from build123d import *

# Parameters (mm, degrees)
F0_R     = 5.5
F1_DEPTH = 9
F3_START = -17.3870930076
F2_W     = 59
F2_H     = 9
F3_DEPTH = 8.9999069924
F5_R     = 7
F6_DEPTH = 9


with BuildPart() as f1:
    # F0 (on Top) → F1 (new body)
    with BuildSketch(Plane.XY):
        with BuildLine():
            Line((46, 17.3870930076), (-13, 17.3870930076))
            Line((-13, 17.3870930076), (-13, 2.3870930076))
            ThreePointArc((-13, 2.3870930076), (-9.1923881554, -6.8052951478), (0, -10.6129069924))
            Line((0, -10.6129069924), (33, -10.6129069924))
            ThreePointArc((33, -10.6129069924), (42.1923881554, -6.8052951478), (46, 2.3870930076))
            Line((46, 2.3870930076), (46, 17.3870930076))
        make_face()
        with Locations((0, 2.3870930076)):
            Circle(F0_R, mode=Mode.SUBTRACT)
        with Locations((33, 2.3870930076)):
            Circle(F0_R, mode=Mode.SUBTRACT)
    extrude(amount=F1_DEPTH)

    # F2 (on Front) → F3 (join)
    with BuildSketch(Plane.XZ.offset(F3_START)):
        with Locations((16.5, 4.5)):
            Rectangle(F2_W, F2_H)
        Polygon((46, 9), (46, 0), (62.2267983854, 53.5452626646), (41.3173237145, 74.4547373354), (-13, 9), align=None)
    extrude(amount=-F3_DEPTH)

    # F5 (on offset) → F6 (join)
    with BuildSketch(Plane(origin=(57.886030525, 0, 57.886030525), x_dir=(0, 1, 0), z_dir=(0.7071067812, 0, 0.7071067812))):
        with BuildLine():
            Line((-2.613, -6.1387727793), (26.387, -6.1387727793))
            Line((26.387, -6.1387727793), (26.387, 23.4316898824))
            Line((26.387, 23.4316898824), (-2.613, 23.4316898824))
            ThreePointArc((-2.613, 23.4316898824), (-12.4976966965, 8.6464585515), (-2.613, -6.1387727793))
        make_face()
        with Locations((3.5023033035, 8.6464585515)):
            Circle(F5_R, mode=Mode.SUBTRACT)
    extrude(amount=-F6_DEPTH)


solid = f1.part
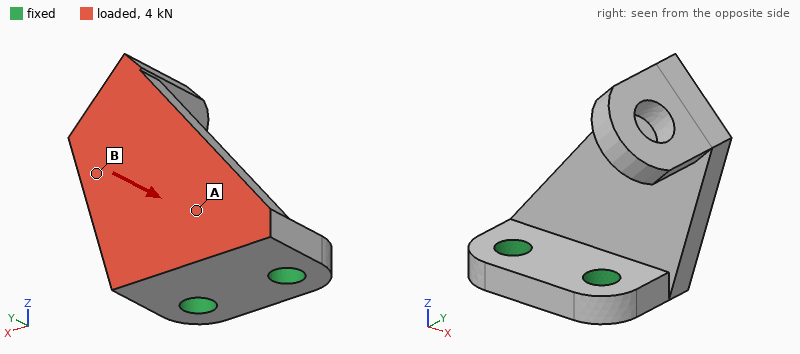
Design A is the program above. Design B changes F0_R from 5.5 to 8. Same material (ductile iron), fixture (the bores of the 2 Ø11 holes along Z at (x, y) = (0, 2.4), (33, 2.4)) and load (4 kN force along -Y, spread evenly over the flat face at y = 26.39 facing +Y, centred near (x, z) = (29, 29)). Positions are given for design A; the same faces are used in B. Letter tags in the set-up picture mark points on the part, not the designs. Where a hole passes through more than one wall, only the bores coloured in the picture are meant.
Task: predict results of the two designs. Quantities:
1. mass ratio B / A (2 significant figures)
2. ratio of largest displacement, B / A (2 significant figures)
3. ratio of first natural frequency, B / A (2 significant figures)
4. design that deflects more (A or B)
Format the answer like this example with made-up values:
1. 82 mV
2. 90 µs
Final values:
1. 0.96
2. 0.92
3. 1.0
4. A
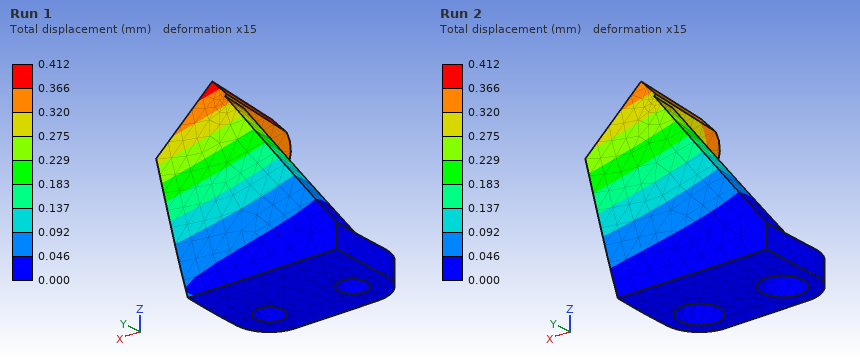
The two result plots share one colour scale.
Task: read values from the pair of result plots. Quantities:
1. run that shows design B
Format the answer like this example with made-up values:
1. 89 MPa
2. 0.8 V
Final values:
1. Run 2
